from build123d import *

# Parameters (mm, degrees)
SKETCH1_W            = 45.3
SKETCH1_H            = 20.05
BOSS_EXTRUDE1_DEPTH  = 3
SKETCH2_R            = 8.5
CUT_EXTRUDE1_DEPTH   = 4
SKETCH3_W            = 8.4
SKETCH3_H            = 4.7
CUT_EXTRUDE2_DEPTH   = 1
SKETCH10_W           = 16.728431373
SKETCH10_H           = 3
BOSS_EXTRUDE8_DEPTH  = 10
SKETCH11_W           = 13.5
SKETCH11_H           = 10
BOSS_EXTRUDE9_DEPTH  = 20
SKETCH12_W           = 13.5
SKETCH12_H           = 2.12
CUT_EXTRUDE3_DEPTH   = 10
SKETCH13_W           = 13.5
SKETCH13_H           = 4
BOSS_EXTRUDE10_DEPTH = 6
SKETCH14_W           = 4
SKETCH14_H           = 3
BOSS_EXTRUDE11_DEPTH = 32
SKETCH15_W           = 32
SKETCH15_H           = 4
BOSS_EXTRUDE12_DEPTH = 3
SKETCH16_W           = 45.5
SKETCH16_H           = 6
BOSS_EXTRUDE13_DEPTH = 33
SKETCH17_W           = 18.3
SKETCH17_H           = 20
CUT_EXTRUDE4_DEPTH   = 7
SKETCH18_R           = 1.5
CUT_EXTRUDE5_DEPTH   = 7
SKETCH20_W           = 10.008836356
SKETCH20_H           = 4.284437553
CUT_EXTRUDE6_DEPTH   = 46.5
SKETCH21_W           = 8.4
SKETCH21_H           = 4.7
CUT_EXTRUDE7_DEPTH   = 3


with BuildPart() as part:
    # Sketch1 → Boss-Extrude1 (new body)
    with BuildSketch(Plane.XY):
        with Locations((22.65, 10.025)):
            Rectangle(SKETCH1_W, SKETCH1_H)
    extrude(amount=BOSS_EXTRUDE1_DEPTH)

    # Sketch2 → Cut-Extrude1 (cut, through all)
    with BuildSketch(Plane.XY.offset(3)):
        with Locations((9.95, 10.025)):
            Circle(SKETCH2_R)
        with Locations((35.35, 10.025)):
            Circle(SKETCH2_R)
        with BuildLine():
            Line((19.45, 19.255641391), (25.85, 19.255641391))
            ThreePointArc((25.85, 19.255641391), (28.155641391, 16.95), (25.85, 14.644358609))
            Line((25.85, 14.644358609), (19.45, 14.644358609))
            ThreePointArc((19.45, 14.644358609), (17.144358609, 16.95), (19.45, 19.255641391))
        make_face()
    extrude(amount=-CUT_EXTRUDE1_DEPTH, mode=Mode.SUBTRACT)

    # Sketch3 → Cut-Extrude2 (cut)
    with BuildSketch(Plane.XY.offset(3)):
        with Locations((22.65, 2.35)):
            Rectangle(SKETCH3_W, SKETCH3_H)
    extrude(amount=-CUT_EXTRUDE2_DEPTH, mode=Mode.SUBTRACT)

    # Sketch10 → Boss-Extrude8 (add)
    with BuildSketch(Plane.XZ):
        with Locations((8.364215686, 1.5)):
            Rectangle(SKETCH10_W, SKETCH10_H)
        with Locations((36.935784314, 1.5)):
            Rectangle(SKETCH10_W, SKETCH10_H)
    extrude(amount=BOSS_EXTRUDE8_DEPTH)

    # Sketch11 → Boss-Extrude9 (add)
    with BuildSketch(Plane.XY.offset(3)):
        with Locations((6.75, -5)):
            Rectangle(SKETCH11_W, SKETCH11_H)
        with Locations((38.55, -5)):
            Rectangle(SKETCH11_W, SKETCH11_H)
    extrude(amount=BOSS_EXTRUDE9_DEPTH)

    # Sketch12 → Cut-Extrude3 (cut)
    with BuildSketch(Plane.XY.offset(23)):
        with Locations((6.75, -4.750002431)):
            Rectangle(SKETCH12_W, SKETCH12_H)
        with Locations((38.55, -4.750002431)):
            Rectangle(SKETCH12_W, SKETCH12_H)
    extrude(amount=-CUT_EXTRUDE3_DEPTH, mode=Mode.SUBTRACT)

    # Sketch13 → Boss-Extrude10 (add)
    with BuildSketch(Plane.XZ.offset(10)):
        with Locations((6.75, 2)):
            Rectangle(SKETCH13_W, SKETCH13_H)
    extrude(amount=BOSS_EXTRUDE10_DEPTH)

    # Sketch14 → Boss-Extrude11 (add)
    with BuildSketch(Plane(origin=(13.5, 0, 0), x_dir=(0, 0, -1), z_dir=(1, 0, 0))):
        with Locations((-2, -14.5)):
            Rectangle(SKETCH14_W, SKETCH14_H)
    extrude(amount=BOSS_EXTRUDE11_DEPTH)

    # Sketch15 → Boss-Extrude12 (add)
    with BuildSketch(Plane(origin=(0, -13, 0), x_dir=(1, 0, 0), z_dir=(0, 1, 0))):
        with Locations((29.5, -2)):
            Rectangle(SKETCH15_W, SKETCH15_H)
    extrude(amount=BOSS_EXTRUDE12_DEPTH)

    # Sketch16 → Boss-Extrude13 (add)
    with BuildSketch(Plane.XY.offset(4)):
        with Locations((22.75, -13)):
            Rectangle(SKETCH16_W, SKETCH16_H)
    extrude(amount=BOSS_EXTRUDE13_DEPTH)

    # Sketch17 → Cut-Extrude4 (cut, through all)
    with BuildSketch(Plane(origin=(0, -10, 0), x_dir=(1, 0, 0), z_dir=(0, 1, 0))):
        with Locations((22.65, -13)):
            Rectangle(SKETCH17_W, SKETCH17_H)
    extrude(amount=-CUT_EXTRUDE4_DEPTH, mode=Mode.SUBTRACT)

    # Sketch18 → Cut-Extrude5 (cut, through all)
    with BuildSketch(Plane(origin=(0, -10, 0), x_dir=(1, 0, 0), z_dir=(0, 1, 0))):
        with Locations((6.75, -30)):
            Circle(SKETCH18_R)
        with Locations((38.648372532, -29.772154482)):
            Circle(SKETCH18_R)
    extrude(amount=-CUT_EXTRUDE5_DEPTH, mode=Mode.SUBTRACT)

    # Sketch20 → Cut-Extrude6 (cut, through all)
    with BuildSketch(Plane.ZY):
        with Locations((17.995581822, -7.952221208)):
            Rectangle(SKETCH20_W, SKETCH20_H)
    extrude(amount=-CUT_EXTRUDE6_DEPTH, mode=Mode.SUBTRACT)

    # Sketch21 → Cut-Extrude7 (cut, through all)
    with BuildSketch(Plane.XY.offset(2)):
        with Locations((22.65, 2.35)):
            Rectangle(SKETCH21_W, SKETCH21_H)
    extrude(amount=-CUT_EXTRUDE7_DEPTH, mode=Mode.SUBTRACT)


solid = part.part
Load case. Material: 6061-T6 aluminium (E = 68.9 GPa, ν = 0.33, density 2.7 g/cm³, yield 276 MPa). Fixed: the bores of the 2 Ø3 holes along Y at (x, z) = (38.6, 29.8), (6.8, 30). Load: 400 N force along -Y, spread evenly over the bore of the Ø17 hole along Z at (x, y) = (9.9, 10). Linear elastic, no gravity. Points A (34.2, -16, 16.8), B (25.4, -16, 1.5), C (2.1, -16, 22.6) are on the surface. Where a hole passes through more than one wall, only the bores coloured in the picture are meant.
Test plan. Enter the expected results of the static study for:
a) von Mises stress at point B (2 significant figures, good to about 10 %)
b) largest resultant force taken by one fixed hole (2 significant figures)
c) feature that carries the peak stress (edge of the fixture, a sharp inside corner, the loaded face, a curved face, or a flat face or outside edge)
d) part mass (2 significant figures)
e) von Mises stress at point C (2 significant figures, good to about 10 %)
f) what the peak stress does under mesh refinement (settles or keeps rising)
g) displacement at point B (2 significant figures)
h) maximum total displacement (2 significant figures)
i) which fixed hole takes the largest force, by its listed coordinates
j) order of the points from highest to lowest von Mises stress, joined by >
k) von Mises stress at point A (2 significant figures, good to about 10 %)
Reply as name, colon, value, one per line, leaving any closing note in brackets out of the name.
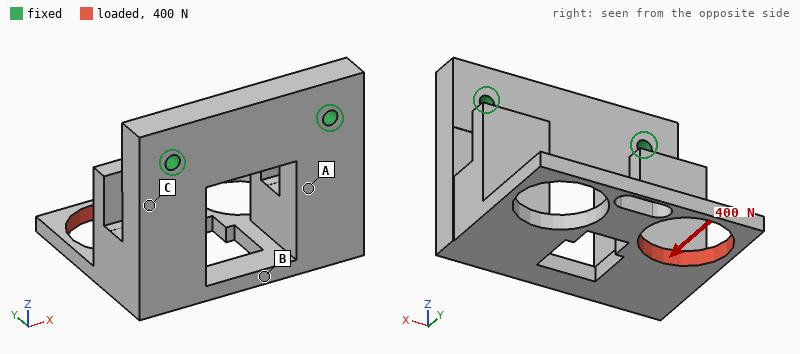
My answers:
von Mises stress at point B: 13 MPa
largest resultant force taken by one fixed hole: 320 N
feature that carries the peak stress: edge of the fixture
part mass: 37 g
von Mises stress at point C: 64 MPa
what the peak stress does under mesh refinement: keeps rising
displacement at point B: 0.088 mm
maximum total displacement: 0.24 mm
which fixed hole takes the largest force, by its listed coordinates: (6.8, 30)
order of the points from highest to lowest von Mises stress, joined by >: C > A > B
von Mises stress at point A: 29 MPa
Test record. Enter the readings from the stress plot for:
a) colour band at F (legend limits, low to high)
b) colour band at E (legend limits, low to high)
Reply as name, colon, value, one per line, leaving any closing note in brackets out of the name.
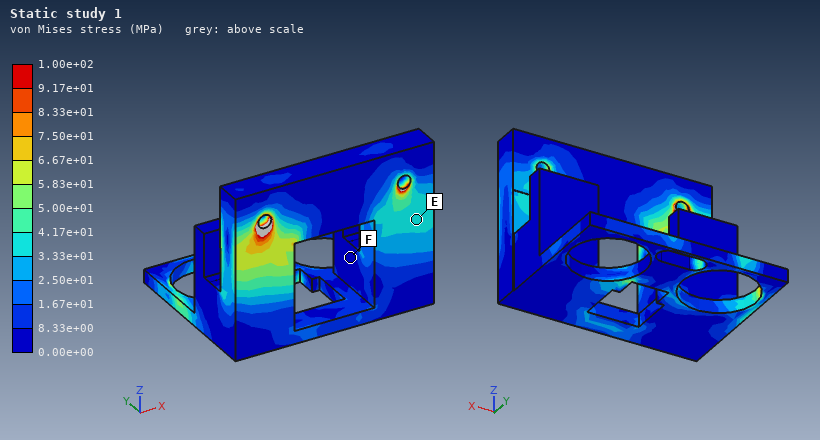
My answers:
colour band at F: 0.00e+00 to 8.33e+00 MPa
colour band at E: 3.33e+01 to 4.17e+01 MPa
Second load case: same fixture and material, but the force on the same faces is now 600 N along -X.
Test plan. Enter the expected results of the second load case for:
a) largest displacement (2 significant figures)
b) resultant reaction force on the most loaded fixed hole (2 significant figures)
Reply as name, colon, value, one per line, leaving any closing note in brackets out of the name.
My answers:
largest displacement: 0.21 mm
resultant reaction force on the most loaded fixed hole: 630 N
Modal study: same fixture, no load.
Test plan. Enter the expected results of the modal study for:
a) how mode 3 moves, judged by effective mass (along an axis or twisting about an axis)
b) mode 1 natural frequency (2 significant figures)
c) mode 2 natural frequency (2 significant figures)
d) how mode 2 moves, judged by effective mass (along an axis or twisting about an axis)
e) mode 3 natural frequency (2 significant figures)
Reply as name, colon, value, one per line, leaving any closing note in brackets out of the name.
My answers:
how mode 3 moves, judged by effective mass: along Y
mode 1 natural frequency: 2200 Hz
mode 2 natural frequency: 3400 Hz
how mode 2 moves, judged by effective mass: along X
mode 3 natural frequency: 4100 Hz
